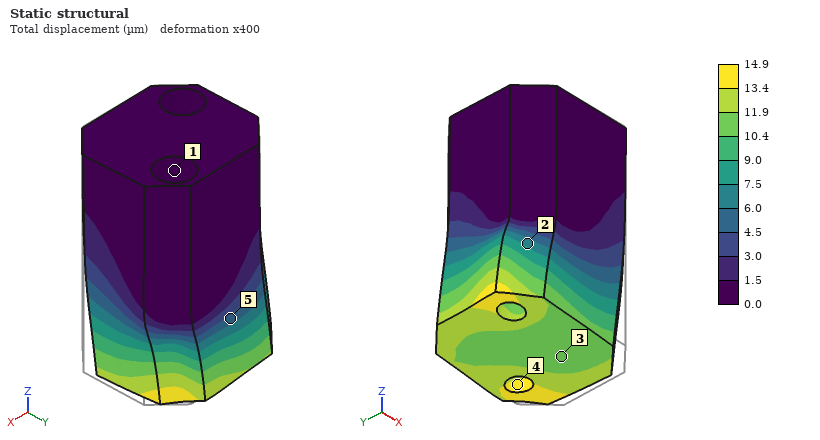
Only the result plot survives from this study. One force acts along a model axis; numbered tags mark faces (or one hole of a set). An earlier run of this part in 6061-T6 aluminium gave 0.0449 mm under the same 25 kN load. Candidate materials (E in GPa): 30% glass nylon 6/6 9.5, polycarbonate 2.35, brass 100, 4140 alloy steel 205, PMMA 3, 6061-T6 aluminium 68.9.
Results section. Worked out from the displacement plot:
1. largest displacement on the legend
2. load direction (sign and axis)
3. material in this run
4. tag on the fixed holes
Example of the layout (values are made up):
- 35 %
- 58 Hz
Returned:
- 14.9 µm
- -X
- 4140 alloy steel
- 1
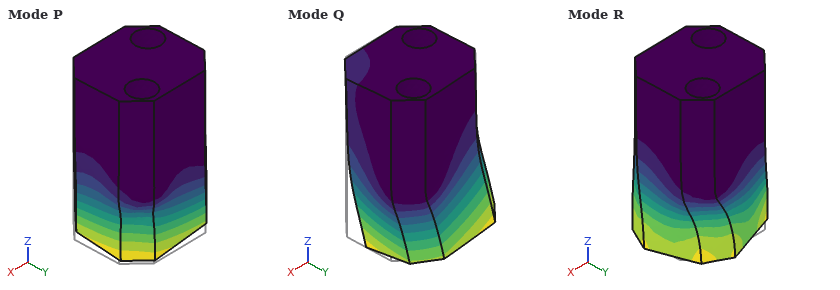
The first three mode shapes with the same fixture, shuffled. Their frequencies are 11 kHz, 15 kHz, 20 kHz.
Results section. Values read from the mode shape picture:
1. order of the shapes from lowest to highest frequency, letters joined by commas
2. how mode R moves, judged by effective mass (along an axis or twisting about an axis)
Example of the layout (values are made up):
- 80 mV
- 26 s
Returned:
- Q, P, R
- twisting about Z
